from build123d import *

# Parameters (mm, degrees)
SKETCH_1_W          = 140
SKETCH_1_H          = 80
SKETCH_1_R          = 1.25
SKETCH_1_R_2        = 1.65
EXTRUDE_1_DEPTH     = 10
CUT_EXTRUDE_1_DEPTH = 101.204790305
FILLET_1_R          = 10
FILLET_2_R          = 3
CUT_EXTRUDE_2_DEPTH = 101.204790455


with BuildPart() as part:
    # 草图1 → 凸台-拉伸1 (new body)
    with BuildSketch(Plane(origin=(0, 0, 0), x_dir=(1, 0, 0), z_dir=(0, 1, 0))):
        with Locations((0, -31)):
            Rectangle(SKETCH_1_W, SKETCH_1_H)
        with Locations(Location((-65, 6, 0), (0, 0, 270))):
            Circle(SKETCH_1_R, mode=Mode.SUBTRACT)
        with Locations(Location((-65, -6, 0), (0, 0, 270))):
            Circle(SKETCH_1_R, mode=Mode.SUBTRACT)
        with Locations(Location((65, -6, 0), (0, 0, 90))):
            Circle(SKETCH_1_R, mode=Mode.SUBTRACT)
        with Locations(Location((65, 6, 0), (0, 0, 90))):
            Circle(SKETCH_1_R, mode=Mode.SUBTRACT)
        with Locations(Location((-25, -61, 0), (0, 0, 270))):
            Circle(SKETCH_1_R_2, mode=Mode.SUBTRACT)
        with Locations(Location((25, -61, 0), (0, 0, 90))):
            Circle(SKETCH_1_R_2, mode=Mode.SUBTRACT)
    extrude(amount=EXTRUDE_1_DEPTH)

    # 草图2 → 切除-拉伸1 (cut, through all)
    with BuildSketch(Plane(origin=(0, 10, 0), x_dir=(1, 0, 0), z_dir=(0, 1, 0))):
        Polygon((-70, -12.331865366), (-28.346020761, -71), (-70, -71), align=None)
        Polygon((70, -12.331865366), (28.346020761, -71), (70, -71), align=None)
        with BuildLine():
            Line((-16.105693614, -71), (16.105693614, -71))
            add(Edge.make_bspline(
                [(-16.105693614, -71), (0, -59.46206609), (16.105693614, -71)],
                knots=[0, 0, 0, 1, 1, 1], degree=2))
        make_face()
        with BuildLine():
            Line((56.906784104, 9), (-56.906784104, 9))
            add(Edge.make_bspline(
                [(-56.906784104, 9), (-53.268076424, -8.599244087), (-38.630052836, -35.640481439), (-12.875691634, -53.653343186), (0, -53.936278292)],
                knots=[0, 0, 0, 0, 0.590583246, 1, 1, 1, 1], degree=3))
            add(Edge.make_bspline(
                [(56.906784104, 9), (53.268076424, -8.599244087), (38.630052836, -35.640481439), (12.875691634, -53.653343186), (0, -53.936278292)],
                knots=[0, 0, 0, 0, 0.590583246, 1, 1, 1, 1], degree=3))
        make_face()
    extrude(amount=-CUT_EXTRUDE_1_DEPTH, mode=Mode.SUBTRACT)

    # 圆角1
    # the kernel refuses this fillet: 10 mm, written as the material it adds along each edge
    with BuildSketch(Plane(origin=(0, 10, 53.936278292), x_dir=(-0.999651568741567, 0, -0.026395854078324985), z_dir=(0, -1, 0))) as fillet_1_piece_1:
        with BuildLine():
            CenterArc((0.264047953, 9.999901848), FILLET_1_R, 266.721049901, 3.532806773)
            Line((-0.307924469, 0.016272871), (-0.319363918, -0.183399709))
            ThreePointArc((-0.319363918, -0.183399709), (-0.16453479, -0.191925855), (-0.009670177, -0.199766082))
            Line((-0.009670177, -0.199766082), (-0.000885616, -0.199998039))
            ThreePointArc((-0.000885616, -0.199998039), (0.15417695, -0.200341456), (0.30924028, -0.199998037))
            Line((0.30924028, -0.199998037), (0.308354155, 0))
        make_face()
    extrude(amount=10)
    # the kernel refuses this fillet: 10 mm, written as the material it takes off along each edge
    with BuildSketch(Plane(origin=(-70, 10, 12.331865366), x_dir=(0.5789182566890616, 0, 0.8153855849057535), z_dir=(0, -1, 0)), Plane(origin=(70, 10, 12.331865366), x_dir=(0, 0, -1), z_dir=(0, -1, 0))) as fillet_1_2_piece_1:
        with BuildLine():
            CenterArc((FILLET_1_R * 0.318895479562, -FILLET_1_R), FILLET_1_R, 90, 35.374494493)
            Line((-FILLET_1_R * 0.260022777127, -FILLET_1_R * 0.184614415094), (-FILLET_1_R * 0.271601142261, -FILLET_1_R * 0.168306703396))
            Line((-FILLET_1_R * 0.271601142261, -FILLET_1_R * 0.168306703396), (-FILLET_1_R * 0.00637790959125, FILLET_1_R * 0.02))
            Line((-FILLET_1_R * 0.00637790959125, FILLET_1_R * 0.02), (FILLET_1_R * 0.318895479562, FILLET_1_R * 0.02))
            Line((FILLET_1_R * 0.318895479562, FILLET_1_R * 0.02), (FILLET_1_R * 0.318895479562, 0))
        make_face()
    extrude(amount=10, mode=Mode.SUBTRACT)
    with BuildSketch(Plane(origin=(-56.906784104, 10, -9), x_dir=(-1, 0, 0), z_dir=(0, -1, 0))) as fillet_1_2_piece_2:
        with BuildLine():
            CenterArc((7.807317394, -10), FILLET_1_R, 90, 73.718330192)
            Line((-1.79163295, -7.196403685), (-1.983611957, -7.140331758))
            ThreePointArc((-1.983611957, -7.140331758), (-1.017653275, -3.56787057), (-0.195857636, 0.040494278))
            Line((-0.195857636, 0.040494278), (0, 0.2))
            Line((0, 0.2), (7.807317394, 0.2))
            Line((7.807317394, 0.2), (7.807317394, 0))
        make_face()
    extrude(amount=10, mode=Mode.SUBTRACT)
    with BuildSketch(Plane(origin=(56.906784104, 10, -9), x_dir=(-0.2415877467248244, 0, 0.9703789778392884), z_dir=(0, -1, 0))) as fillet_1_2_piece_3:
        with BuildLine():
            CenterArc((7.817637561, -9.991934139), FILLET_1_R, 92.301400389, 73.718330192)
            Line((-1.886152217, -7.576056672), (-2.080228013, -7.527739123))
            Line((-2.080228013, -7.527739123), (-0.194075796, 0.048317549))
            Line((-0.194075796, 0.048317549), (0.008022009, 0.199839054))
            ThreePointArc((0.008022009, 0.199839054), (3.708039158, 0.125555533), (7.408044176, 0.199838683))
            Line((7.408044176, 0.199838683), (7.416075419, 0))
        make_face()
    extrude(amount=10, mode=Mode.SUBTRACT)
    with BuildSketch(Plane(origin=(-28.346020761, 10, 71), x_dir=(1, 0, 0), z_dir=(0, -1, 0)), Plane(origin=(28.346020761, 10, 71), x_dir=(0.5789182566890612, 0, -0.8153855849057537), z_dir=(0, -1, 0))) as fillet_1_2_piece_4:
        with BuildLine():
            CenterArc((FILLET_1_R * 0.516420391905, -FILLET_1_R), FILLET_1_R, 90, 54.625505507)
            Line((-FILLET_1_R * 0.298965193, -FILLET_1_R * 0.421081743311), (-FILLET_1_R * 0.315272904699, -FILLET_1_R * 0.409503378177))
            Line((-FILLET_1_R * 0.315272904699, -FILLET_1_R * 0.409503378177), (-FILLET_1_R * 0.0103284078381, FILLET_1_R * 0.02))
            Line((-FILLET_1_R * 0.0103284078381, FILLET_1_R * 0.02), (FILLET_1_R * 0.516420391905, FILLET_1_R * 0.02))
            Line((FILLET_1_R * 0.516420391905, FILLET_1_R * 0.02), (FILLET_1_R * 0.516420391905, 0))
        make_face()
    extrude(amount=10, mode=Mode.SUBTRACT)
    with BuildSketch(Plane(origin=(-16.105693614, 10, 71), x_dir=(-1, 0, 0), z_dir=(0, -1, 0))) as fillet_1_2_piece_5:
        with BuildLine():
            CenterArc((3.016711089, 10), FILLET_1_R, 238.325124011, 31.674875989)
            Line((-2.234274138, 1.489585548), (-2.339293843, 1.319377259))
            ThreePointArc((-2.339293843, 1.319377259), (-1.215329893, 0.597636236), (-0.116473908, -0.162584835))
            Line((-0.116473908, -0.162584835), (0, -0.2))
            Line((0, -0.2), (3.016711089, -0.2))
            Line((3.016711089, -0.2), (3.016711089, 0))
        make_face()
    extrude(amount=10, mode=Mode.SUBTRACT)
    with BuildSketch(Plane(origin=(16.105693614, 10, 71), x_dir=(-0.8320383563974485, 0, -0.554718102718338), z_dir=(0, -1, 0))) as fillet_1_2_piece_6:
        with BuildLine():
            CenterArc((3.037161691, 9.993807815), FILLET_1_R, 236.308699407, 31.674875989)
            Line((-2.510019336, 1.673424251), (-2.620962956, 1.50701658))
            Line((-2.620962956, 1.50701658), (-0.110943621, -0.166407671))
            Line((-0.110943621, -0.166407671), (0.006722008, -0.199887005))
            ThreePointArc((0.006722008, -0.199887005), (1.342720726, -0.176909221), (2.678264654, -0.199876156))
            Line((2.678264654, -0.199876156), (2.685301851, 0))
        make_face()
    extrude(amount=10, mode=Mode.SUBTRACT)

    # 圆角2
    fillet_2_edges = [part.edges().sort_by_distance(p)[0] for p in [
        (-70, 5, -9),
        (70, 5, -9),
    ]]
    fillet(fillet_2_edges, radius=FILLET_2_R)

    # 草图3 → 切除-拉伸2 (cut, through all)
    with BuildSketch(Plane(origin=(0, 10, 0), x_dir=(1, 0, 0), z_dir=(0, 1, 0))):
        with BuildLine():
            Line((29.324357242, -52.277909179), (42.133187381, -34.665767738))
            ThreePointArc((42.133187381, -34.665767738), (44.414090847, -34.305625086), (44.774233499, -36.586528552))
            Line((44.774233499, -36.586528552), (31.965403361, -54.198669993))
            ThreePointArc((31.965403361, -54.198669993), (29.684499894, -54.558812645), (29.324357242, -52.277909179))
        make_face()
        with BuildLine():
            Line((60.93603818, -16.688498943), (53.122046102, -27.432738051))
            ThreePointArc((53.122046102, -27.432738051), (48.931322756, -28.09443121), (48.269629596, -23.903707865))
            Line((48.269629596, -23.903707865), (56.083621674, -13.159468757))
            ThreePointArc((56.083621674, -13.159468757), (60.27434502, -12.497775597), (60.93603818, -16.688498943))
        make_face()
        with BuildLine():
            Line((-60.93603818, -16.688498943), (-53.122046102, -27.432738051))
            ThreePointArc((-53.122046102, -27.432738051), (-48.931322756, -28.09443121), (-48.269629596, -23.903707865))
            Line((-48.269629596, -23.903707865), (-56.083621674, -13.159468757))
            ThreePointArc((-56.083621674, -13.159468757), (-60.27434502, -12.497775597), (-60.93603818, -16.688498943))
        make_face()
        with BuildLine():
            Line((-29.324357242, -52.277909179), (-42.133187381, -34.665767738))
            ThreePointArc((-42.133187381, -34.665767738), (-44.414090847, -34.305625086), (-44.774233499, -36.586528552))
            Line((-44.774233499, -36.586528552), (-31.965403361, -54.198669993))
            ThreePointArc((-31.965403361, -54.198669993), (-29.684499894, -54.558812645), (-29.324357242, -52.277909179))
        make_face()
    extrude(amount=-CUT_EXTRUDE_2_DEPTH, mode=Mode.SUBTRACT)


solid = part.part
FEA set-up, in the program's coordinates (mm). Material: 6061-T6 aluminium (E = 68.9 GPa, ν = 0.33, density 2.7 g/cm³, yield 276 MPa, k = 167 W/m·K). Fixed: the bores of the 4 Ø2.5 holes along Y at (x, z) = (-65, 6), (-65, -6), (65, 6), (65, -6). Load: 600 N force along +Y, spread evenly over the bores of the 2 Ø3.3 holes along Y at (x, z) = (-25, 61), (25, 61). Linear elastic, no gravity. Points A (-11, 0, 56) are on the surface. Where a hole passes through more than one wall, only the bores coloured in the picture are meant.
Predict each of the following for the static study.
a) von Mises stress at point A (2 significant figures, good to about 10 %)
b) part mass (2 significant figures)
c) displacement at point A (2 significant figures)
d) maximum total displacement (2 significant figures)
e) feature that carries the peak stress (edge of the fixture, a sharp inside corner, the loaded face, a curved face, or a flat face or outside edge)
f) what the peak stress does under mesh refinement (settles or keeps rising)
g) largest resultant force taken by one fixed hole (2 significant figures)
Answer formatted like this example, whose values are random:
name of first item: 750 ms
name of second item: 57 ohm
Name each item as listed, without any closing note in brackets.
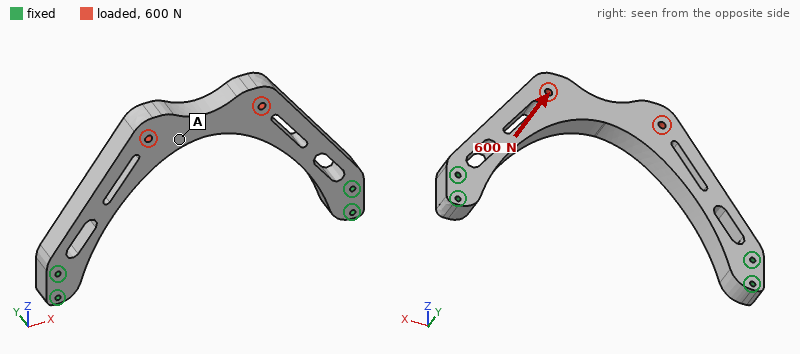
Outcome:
von Mises stress at point A: 15 MPa
part mass: 83 g
displacement at point A: 0.38 mm
maximum total displacement: 0.51 mm
feature that carries the peak stress: edge of the fixture
what the peak stress does under mesh refinement: keeps rising
largest resultant force taken by one fixed hole: 760 N
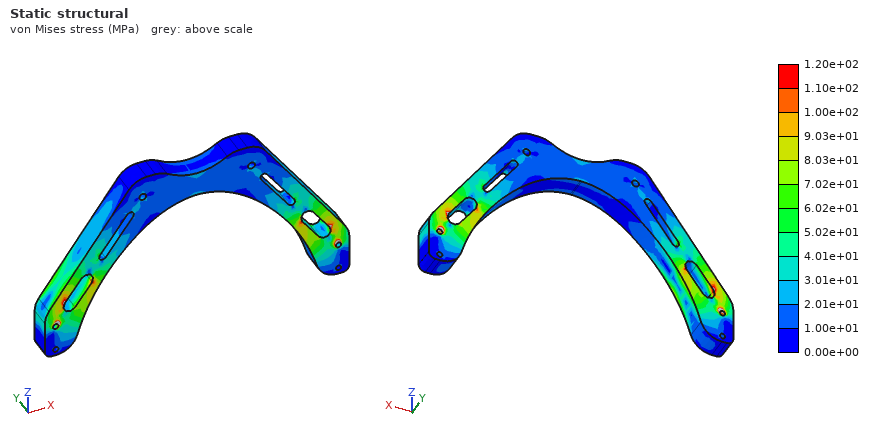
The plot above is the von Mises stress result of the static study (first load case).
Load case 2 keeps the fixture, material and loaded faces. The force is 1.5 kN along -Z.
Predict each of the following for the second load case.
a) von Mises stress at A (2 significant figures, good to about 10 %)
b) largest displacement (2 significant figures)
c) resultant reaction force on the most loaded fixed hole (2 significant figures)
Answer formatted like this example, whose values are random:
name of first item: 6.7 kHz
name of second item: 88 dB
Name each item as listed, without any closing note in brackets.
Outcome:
von Mises stress at A: 2.8 MPa
largest displacement: 12 µm
resultant reaction force on the most loaded fixed hole: 670 N
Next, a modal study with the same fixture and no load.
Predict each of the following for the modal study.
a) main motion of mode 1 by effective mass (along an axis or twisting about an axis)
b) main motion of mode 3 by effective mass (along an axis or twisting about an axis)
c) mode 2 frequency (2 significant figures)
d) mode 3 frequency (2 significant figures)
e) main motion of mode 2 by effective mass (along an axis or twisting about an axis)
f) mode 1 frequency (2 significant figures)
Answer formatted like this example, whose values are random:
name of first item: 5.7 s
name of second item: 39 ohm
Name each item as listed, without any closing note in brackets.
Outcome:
main motion of mode 1 by effective mass: along Y
main motion of mode 3 by effective mass: along X
mode 2 frequency: 3000 Hz
mode 3 frequency: 3800 Hz
main motion of mode 2 by effective mass: twisting about Z
mode 1 frequency: 980 Hz
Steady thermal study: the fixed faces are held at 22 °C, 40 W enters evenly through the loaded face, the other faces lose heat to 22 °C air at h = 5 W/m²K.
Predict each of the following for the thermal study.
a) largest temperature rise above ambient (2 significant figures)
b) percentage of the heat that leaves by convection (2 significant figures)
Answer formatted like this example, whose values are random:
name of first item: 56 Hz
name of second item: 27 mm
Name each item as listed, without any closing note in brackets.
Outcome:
largest temperature rise above ambient: 62 K
percentage of the heat that leaves by convection: 5.4 %
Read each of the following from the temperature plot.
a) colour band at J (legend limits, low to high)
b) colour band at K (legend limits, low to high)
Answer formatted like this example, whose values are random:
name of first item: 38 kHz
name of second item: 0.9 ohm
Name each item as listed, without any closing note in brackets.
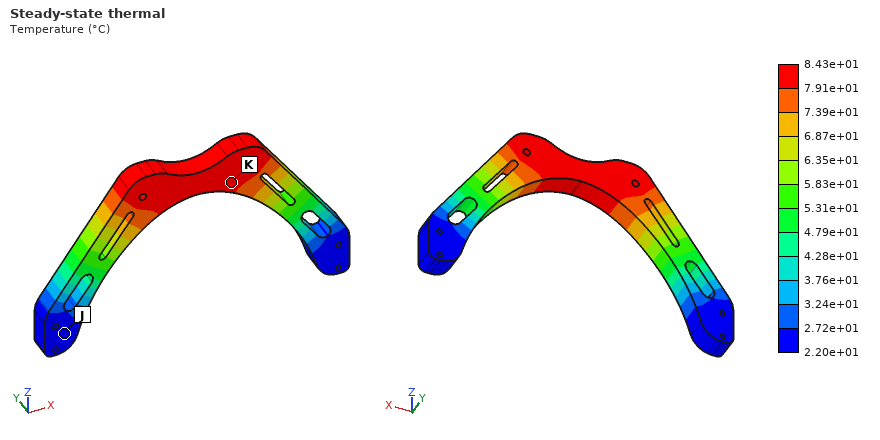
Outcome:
colour band at J: 2.20e+01 to 2.72e+01 °C
colour band at K: 7.91e+01 to 8.43e+01 °C
